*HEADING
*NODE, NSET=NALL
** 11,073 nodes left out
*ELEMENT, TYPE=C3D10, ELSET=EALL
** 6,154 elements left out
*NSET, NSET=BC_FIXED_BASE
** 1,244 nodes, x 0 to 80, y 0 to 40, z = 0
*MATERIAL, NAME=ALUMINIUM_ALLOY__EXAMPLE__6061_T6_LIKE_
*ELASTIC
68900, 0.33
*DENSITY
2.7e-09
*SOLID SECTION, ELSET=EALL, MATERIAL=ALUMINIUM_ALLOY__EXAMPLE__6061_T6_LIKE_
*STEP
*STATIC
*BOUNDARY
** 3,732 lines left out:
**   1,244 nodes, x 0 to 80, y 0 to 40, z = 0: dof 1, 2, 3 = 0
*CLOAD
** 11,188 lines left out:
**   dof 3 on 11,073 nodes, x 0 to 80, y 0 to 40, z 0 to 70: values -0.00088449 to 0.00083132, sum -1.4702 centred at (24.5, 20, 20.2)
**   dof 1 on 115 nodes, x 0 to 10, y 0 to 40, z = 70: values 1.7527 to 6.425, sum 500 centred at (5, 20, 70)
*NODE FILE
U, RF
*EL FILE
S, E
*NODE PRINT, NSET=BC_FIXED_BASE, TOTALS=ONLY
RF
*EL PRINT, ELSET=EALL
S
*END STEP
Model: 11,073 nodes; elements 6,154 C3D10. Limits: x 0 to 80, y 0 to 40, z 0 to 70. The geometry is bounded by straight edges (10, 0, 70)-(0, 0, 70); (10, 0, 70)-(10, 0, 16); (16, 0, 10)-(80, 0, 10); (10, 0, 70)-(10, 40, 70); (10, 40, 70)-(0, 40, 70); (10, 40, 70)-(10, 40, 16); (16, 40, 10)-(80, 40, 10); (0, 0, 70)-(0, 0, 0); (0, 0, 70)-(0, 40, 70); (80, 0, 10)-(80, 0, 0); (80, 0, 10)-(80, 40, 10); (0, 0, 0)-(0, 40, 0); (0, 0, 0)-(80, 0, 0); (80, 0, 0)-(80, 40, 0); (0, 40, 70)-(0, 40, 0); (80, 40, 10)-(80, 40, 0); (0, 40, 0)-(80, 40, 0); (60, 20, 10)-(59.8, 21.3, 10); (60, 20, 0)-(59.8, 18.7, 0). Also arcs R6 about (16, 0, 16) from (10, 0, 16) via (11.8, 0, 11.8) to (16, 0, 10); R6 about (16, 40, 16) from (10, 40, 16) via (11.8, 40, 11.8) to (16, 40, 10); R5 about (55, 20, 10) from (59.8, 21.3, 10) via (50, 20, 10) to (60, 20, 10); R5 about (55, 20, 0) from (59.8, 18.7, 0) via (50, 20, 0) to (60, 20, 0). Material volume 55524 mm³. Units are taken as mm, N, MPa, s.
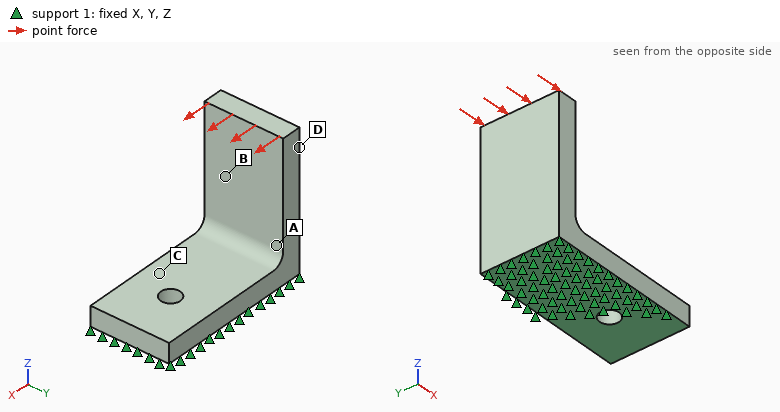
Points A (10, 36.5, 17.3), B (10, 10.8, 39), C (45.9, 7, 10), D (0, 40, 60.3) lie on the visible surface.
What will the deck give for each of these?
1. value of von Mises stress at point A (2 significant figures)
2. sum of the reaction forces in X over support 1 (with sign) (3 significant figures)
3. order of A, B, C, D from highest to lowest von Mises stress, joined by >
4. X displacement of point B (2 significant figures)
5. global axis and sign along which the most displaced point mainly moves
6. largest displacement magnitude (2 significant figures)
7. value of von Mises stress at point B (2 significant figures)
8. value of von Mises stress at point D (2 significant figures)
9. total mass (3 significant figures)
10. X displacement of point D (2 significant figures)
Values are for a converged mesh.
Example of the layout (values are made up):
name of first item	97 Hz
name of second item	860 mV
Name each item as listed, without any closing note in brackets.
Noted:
value of von Mises stress at point A	40 MPa
sum of the reaction forces in X over support 1 (with sign)	-500 N
order of A, B, C, D from highest to lowest von Mises stress, joined by >	A > B > D > C
X displacement of point B	0.054 mm
global axis and sign along which the most displaced point mainly moves	+X
largest displacement magnitude	0.17 mm
value of von Mises stress at point B	23 MPa
value of von Mises stress at point D	7.3 MPa
total mass	0.150 kg
X displacement of point D	0.13 mm
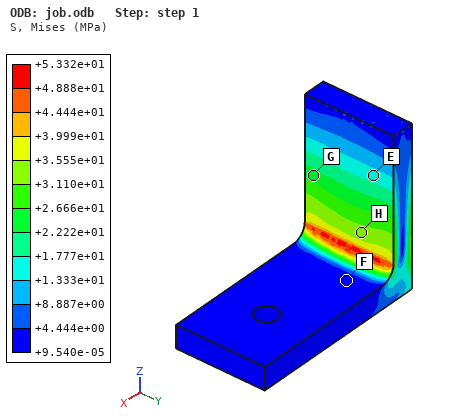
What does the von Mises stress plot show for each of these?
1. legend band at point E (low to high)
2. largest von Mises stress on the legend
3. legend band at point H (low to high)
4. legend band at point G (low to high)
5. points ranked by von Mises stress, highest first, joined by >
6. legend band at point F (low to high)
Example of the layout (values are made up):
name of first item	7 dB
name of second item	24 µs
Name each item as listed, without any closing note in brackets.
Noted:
legend band at point E	+1.333e+01 to +1.777e+01 MPa
largest von Mises stress on the legend	+5.332e+01 MPa
legend band at point H	+3.110e+01 to +3.555e+01 MPa
legend band at point G	+2.222e+01 to +2.666e+01 MPa
points ranked by von Mises stress, highest first, joined by >	H > G > E > F
legend band at point F	+9.540e-05 to +4.444e+00 MPa
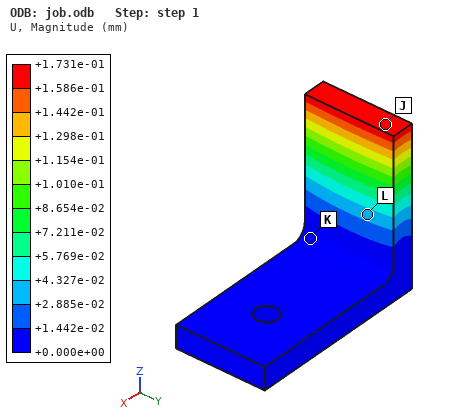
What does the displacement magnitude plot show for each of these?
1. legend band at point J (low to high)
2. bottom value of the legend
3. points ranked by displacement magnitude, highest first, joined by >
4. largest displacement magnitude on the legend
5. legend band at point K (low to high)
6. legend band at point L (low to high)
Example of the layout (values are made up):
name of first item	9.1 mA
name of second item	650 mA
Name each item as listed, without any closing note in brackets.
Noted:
legend band at point J	+1.586e-01 to +1.731e-01 mm
bottom value of the legend	+0.000e+00 mm
points ranked by displacement magnitude, highest first, joined by >	J > L > K
largest displacement magnitude on the legend	+1.731e-01 mm
legend band at point K	+0.000e+00 to +1.442e-02 mm
legend band at point L	+2.885e-02 to +4.327e-02 mm
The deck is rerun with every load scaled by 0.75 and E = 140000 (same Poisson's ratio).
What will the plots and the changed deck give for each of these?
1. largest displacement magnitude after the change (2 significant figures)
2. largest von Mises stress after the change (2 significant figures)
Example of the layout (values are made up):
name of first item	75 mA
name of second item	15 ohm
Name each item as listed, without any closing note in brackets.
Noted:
largest displacement magnitude after the change	0.064 mm
largest von Mises stress after the change	40 MPa
